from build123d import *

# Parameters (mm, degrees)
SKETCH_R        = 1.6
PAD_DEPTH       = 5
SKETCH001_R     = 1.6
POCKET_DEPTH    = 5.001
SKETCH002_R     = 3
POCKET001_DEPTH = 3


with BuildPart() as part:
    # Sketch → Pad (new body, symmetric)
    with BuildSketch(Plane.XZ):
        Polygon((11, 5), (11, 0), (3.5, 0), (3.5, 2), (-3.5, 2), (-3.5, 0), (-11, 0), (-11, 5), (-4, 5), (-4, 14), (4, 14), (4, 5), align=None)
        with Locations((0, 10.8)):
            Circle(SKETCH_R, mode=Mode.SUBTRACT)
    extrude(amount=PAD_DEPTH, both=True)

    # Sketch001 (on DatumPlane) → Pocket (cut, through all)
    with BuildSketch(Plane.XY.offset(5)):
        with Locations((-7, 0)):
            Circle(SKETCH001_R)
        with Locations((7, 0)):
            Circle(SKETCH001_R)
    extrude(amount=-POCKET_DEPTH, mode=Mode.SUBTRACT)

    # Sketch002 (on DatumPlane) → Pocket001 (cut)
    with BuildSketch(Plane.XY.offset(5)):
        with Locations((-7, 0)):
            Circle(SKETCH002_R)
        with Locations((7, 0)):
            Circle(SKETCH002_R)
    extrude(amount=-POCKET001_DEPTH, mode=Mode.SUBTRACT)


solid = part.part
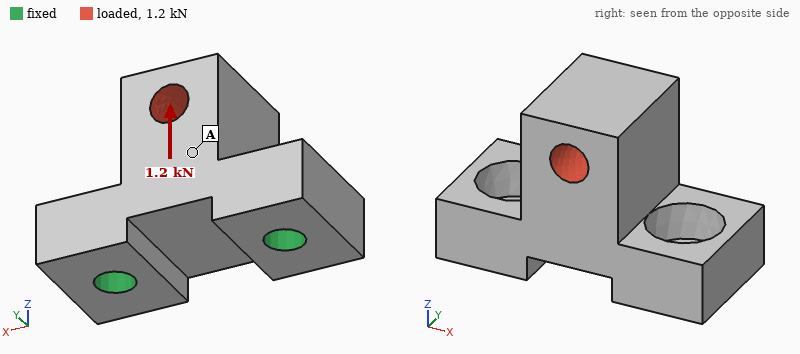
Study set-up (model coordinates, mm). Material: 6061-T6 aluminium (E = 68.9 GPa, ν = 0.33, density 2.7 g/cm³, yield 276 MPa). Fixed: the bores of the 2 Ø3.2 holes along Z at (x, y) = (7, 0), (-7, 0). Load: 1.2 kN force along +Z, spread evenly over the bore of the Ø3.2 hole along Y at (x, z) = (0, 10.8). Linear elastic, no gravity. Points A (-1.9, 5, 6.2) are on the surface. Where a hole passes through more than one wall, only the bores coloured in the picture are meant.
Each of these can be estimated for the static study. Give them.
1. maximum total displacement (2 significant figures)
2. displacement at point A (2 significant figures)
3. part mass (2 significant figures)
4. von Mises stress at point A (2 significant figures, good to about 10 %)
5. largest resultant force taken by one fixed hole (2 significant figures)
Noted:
9.3 µm
6.7 µm
3.8 g
18 MPa
710 N
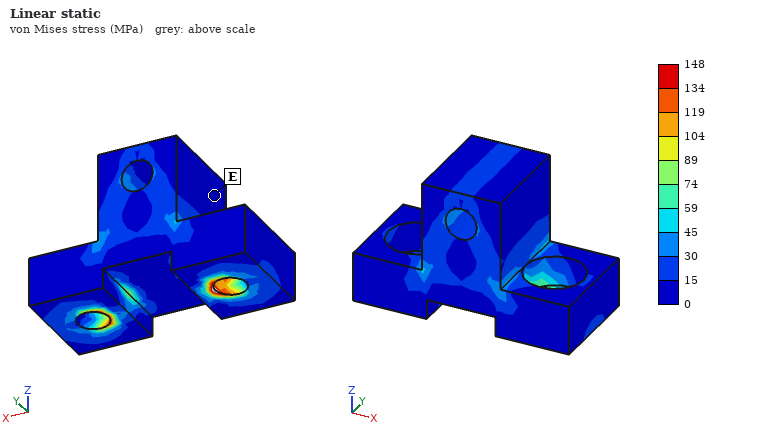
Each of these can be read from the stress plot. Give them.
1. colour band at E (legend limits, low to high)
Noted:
0 to 15 MPa
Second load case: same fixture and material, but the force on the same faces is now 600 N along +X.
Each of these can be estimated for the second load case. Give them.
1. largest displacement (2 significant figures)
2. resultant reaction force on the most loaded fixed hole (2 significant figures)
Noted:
19 µm
570 N
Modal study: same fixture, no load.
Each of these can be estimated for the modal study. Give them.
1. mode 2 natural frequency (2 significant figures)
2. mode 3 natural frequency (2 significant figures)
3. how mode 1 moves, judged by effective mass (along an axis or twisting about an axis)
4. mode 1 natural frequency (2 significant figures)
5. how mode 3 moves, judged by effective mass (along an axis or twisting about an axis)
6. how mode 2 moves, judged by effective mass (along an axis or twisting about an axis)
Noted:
28 kHz
41 kHz
along Y
13 kHz
along Z
along X
